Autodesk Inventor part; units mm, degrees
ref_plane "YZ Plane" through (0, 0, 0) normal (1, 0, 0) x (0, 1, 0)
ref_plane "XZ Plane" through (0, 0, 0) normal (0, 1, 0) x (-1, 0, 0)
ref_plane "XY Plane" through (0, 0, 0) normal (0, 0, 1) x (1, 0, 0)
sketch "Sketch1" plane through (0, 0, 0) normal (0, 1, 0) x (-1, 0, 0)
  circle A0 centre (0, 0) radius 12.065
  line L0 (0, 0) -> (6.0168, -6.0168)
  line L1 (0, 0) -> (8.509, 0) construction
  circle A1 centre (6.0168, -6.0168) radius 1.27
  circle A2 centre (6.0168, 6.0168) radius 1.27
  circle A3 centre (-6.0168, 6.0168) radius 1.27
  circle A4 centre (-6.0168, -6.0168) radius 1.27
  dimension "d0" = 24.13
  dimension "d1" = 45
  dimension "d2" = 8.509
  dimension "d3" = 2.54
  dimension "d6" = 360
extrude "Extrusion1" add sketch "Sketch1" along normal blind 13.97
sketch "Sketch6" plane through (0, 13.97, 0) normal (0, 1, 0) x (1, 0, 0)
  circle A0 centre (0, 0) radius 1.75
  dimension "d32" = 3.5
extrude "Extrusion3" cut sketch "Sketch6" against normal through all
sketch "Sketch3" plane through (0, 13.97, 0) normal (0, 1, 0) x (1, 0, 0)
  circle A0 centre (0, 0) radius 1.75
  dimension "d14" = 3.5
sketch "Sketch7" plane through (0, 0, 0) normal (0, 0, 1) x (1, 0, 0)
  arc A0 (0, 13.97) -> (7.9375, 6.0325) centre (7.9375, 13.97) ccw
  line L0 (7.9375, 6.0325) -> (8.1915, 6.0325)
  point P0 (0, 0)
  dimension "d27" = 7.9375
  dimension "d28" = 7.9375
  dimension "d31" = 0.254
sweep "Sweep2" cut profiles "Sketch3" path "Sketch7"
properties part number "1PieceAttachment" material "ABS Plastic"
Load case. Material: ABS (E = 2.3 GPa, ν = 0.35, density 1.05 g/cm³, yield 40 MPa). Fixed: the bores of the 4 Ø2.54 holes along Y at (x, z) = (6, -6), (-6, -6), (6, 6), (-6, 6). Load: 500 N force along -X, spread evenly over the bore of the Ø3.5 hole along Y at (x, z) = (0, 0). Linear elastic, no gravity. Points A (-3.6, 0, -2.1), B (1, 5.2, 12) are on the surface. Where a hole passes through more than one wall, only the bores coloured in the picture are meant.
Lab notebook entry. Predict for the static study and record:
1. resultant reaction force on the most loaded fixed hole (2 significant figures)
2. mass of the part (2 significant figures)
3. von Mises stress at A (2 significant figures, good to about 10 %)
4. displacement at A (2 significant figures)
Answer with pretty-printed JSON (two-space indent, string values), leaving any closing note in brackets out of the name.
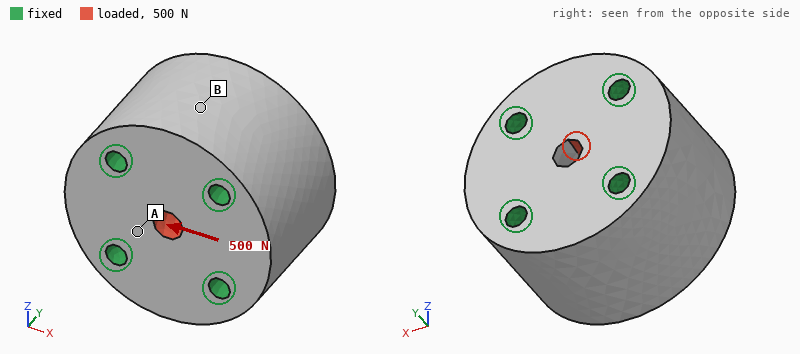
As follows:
{
  "resultant reaction force on the most loaded fixed hole": "150 N",
  "mass of the part": "6.2 g",
  "von Mises stress at A": "2.7 MPa",
  "displacement at A": "5.6 µm"
}
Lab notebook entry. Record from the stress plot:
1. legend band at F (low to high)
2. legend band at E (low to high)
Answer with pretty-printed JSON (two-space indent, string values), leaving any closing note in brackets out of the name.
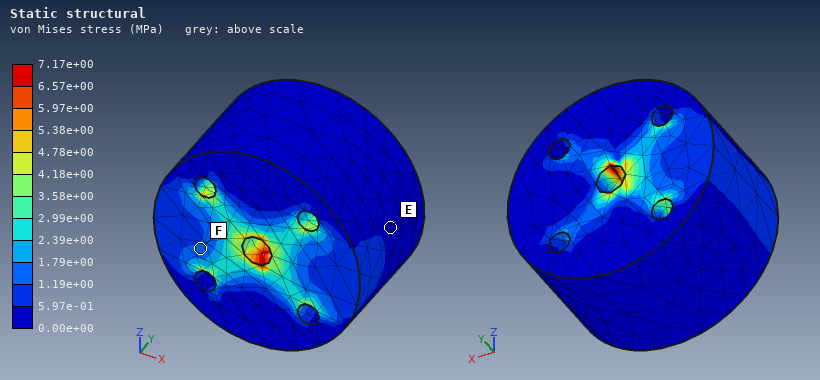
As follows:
{
  "legend band at F": "1.19e+00 to 1.79e+00 MPa",
  "legend band at E": "0.00e+00 to 5.97e-01 MPa"
}
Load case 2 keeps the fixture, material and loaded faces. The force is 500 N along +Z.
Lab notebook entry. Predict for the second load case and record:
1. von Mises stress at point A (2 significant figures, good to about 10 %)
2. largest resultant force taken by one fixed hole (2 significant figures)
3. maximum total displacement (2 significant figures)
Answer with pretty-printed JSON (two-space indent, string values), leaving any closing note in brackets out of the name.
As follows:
{
  "von Mises stress at point A": "2.2 MPa",
  "largest resultant force taken by one fixed hole": "150 N",
  "maximum total displacement": "10 µm"
}
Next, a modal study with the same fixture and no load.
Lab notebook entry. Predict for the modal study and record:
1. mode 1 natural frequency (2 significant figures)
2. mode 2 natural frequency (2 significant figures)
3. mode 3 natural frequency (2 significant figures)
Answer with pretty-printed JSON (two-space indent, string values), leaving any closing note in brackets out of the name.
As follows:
{
  "mode 1 natural frequency": "30 kHz",
  "mode 2 natural frequency": "30 kHz",
  "mode 3 natural frequency": "30 kHz"
}
